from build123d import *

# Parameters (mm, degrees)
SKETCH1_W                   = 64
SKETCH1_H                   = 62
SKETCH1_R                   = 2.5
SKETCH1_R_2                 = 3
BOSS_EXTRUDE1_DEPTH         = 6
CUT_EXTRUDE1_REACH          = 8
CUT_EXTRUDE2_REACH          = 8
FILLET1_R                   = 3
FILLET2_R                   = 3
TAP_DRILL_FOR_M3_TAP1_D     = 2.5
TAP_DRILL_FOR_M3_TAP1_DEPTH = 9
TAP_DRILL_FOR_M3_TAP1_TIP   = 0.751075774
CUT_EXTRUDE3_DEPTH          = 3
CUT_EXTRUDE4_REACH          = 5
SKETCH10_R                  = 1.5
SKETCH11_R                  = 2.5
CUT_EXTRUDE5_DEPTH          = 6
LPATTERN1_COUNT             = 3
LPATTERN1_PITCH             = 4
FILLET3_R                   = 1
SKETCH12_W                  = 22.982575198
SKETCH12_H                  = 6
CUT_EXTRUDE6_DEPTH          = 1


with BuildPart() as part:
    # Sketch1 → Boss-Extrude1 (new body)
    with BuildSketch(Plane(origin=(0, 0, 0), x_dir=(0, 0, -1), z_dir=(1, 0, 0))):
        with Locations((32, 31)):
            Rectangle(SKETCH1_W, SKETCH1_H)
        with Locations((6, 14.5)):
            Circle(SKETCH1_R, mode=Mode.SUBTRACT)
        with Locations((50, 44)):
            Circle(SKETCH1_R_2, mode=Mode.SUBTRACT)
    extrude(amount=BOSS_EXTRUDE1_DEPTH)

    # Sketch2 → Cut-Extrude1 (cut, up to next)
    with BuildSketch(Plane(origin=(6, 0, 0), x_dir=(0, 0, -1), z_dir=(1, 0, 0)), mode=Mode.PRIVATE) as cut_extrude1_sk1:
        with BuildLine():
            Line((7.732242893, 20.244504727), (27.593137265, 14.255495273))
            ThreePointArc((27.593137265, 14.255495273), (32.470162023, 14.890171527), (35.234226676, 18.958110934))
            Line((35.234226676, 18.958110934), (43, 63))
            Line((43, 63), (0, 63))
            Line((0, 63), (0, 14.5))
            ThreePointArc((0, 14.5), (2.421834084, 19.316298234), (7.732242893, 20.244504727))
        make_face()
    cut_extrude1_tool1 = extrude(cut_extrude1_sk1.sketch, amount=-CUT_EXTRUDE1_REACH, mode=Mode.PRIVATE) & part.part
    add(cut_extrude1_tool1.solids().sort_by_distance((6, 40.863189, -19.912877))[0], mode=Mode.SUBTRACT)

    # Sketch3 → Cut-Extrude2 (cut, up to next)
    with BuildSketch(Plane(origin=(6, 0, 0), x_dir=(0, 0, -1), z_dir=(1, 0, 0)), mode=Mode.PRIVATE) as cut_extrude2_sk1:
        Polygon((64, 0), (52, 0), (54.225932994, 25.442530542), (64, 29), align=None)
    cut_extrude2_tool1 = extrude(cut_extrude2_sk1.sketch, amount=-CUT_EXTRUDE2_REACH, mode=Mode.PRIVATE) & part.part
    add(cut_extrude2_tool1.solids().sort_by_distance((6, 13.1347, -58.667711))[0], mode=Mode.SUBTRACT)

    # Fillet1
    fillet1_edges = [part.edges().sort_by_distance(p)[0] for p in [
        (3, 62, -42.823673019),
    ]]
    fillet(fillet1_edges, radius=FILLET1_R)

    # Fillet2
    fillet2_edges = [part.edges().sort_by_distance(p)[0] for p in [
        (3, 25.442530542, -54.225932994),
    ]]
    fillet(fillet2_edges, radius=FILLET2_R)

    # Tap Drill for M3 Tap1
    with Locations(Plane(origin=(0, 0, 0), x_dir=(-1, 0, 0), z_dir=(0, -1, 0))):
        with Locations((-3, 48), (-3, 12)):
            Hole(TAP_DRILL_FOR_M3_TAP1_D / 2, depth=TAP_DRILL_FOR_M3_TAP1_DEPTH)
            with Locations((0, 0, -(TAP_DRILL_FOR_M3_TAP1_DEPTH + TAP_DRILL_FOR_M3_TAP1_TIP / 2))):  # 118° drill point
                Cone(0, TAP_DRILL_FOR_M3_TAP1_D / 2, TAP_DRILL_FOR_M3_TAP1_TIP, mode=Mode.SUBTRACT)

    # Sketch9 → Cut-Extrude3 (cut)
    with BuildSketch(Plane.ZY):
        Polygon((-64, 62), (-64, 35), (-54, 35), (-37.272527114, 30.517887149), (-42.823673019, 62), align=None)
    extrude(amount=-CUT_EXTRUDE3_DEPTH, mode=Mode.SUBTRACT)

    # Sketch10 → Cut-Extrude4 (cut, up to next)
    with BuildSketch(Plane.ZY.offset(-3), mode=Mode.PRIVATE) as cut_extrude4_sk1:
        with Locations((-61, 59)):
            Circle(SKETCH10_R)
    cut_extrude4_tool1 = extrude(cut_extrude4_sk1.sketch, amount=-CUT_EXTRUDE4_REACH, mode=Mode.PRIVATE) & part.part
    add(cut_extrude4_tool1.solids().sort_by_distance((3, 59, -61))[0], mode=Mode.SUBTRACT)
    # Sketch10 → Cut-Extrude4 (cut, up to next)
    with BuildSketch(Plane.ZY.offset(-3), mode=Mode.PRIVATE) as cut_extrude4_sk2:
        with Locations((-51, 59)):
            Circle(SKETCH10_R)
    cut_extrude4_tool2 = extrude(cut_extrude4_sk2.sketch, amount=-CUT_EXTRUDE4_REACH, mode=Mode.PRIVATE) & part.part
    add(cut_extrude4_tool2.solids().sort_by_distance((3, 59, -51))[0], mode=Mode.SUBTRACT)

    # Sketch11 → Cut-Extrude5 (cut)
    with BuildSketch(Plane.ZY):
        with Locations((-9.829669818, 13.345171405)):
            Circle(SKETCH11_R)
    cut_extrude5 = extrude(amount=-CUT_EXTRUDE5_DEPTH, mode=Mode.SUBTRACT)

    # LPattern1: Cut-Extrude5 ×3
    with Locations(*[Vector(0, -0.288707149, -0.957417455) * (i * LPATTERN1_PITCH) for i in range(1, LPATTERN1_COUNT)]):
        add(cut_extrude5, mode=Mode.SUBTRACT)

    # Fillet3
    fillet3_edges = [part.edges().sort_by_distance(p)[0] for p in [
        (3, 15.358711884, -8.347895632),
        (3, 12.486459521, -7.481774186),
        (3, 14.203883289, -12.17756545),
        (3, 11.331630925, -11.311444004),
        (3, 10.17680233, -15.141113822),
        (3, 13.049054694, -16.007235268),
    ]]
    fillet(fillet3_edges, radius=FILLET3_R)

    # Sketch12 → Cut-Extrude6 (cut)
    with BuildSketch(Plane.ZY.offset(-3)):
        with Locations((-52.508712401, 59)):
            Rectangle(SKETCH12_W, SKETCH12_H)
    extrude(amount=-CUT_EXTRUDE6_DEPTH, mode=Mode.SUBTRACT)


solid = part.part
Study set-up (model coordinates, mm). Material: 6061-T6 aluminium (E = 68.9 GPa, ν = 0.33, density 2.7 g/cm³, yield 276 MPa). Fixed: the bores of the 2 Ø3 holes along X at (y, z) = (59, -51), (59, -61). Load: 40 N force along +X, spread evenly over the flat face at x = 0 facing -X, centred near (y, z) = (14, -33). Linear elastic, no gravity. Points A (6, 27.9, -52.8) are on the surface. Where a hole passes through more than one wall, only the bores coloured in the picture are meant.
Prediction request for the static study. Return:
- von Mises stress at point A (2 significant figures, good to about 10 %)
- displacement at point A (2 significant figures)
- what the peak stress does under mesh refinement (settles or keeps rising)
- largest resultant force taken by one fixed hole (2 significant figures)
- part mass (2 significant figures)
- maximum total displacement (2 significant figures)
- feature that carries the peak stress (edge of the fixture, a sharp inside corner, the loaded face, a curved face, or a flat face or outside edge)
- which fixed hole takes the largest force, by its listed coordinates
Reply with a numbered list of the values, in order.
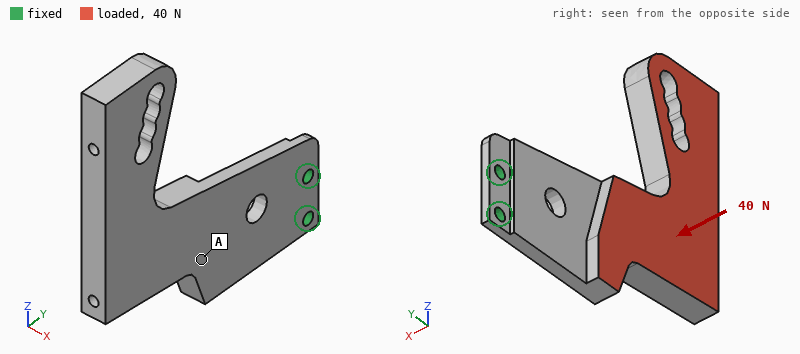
1. 12 MPa
2. 0.31 mm
3. keeps rising
4. 99 N
5. 24 g
6. 0.96 mm
7. edge of the fixture
8. (59, -51)
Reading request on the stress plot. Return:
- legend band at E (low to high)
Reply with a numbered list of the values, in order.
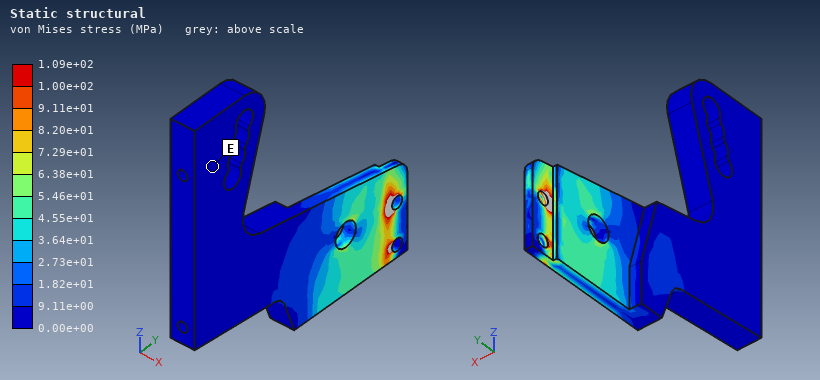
1. 0.00e+00 to 9.11e+00 MPa
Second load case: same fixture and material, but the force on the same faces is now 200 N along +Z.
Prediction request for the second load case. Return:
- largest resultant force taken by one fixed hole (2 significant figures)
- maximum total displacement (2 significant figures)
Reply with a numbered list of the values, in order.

1. 780 N
2. 0.23 mm
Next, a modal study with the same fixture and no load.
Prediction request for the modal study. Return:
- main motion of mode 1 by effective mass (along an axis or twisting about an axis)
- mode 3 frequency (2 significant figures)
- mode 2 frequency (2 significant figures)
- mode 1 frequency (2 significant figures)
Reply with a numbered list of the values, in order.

1. along X
2. 1600 Hz
3. 1100 Hz
4. 280 Hz
